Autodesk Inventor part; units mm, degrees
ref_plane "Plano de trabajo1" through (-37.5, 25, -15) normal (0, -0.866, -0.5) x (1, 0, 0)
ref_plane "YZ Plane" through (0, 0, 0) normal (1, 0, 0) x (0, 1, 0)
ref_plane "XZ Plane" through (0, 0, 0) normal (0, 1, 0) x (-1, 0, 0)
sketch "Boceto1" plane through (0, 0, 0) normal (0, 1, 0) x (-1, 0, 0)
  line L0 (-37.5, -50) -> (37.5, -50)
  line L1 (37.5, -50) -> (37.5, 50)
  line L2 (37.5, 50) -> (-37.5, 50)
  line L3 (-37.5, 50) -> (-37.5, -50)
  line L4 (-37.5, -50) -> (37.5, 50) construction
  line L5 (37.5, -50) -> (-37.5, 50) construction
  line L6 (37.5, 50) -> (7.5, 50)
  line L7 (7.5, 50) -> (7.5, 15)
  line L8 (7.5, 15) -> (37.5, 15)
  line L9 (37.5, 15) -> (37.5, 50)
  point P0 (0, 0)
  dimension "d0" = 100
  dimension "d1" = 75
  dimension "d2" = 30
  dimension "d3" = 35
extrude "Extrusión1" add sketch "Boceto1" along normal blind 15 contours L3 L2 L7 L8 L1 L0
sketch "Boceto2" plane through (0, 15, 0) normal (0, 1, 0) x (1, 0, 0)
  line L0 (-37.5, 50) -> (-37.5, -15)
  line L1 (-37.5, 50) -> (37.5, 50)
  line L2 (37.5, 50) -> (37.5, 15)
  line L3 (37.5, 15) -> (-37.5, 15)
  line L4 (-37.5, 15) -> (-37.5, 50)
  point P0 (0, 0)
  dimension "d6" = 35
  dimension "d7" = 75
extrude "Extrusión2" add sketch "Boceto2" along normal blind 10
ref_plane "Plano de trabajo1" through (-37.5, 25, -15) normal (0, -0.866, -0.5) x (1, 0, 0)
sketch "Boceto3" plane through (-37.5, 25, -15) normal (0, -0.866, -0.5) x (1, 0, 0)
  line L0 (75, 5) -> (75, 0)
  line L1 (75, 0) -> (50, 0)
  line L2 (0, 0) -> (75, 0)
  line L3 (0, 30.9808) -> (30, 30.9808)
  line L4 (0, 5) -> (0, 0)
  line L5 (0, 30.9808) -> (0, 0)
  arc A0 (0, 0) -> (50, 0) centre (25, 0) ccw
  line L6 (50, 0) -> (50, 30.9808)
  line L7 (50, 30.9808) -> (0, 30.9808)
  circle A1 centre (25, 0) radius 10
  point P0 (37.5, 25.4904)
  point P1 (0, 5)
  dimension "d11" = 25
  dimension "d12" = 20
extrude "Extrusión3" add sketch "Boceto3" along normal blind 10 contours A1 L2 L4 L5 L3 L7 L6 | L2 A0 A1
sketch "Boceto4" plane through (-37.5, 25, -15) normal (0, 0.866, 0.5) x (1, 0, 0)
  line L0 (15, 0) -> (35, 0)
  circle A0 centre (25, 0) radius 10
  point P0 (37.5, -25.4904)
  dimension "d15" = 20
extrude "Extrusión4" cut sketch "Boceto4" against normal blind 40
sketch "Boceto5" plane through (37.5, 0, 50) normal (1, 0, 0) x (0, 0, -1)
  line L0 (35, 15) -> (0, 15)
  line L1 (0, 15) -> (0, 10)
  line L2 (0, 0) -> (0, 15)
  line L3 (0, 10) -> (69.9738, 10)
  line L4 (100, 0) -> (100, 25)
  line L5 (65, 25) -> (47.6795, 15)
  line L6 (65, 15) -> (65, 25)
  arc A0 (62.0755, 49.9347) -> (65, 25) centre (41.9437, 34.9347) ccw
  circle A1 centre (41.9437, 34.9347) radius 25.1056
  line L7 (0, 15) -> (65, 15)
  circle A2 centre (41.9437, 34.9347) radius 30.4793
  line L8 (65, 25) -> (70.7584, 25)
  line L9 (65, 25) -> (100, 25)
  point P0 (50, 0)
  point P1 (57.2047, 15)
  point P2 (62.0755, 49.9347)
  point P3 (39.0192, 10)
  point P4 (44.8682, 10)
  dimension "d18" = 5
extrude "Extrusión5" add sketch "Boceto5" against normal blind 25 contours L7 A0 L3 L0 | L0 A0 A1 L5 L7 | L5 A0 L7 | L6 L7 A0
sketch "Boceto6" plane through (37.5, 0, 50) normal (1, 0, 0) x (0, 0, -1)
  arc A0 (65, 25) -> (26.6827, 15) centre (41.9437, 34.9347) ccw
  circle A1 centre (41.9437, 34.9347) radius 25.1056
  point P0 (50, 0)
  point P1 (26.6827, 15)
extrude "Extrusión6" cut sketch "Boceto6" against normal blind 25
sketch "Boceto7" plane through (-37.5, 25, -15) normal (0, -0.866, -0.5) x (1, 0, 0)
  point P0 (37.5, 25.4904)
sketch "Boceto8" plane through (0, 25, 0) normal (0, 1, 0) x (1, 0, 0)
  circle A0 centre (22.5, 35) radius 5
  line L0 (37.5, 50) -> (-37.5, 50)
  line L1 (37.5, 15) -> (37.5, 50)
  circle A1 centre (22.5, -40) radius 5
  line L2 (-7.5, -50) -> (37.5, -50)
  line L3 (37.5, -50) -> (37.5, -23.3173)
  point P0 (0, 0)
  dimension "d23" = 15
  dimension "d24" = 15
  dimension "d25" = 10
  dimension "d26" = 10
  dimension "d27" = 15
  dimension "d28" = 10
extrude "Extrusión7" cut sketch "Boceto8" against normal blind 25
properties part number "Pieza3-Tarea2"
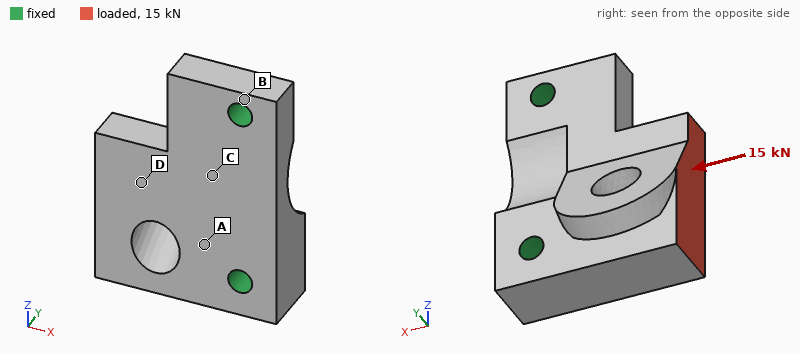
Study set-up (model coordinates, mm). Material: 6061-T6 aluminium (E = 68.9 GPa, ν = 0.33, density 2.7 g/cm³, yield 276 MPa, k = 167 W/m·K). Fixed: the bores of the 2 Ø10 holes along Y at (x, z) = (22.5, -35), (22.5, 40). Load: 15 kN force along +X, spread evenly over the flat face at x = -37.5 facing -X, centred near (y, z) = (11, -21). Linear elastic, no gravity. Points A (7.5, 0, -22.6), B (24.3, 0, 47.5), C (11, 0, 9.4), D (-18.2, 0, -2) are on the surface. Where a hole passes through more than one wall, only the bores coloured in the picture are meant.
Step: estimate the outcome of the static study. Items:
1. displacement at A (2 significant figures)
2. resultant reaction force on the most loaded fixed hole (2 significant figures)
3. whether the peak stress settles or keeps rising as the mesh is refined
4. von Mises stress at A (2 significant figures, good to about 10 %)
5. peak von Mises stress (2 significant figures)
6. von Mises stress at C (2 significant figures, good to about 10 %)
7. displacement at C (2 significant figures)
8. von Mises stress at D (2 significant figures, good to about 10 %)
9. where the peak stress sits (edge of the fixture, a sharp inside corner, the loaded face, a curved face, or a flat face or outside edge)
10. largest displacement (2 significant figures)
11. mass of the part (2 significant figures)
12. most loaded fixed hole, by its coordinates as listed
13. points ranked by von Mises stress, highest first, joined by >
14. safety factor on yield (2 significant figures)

4.3 µm
12 kN
settles
18 MPa
46 MPa
7.9 MPa
8.4 µm
11 MPa
a curved face
20 µm
320 g
(22.5, -35)
A > D > C > B
6.0
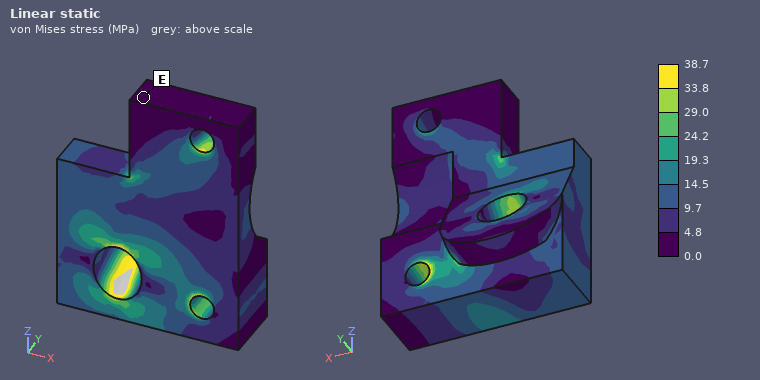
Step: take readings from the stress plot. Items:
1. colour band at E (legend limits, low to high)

0.0 to 4.8 MPa
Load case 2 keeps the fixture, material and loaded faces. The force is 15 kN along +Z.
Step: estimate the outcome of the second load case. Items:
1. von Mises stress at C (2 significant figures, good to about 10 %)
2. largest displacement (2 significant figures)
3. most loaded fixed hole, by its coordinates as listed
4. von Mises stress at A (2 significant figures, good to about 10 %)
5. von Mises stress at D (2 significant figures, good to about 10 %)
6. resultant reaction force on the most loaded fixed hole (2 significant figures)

14 MPa
97 µm
(22.5, 40)
29 MPa
53 MPa
14 kN
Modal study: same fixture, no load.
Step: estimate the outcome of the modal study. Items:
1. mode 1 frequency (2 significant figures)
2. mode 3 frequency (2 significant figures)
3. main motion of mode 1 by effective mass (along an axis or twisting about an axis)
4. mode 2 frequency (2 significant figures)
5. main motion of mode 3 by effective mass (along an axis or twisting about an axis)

4100 Hz
8500 Hz
along Y
7600 Hz
along Z
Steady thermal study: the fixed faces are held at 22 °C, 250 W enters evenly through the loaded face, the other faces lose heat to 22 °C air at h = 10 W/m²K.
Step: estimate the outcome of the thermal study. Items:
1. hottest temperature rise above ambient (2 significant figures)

76 K
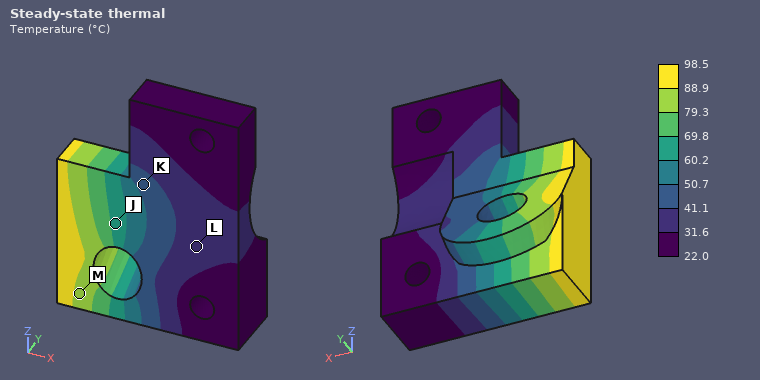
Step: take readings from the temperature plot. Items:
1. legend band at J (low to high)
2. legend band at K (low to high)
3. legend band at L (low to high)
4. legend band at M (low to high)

60.2 to 69.8 °C
41.1 to 50.7 °C
31.6 to 41.1 °C
79.3 to 88.9 °C
